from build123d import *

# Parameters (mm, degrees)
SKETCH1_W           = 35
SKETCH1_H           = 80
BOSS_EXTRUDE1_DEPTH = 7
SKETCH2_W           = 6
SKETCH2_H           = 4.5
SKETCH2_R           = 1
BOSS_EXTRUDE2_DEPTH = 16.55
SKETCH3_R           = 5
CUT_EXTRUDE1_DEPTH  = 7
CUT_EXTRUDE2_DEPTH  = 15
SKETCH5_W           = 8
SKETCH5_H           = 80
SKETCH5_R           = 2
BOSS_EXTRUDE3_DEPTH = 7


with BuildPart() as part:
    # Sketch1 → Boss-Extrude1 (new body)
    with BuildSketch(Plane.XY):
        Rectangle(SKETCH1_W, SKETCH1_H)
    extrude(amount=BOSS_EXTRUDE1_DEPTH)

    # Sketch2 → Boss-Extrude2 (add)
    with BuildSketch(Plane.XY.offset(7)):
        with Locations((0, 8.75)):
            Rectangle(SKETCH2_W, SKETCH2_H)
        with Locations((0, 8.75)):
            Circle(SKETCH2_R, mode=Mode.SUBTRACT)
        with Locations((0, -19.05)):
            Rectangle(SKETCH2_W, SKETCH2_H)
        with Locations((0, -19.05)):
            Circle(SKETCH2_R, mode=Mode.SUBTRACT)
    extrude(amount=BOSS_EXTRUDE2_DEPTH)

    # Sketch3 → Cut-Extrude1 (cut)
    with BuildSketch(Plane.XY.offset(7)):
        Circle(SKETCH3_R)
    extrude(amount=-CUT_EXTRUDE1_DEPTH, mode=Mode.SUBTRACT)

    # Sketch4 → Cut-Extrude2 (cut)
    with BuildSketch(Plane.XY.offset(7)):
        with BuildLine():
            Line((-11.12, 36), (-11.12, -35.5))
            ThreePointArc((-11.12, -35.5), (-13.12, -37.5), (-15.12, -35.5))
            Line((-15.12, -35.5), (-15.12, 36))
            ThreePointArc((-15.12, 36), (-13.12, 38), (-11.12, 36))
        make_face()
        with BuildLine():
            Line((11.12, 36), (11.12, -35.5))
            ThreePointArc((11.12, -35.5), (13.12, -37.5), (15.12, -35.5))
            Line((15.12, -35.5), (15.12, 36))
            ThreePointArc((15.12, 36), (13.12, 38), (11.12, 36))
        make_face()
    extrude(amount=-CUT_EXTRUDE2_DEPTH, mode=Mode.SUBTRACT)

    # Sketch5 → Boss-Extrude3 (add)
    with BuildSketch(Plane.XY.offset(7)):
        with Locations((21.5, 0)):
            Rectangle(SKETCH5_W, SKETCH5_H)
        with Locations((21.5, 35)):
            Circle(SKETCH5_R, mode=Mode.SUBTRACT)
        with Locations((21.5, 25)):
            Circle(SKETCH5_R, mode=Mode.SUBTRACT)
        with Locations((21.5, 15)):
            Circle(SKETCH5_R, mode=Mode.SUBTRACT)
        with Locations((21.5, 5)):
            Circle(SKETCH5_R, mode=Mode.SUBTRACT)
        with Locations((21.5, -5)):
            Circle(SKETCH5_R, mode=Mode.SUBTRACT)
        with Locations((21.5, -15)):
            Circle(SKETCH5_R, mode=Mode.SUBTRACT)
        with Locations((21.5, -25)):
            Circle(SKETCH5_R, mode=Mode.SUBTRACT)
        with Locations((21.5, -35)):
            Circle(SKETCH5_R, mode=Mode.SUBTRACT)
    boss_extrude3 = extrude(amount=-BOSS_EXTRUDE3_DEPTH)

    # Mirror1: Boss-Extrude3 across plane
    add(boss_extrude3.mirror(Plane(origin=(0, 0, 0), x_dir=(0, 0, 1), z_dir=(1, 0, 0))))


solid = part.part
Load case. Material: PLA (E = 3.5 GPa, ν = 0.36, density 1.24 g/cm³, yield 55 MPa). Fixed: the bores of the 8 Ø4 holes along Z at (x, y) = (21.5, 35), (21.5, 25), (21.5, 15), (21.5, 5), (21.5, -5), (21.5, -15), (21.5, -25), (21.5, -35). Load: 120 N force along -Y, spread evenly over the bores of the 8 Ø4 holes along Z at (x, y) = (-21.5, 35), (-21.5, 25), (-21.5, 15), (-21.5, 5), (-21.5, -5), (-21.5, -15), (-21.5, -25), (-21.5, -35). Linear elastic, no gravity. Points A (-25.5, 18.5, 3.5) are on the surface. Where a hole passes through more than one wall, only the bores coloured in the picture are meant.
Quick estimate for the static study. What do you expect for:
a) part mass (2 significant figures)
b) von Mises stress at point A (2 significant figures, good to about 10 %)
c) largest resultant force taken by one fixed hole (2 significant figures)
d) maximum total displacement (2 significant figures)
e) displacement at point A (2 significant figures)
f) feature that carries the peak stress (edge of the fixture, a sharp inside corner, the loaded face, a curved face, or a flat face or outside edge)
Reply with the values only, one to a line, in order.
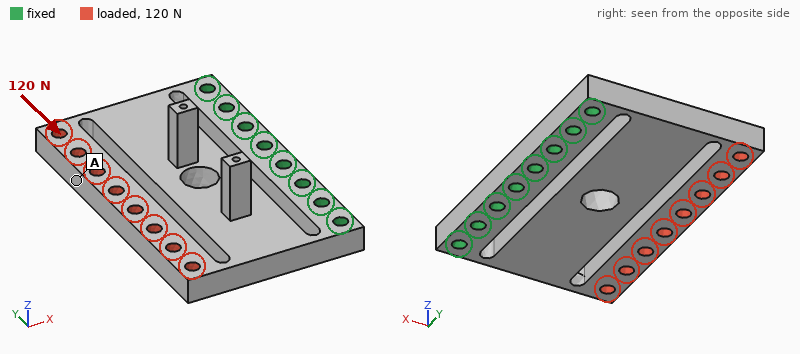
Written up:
29 g
1.3 MPa
85 N
0.17 mm
0.15 mm
a curved face
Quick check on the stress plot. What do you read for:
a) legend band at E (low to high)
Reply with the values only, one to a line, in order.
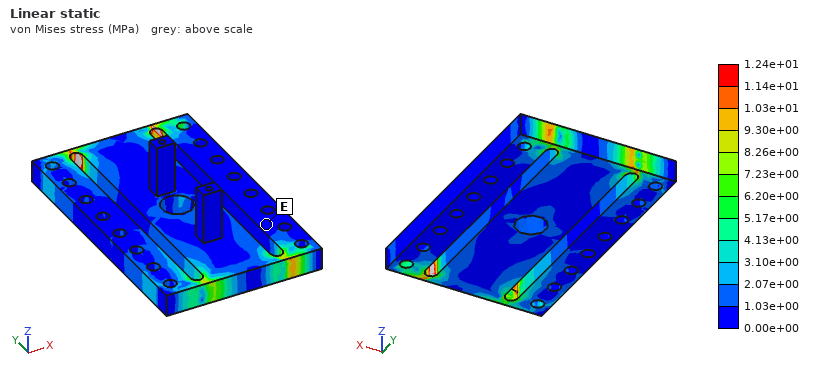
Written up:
0.00e+00 to 1.03e+00 MPa
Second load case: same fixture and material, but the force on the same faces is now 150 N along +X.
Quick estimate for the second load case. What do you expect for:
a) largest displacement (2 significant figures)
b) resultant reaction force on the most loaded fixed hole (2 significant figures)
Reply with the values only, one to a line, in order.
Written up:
0.32 mm
82 N
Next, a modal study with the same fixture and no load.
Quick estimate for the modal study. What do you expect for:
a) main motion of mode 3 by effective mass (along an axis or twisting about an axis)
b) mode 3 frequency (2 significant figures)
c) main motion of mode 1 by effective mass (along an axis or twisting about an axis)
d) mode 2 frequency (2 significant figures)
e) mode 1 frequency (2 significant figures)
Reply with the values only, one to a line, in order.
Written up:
twisting about X
1000 Hz
along Z
920 Hz
300 Hz
